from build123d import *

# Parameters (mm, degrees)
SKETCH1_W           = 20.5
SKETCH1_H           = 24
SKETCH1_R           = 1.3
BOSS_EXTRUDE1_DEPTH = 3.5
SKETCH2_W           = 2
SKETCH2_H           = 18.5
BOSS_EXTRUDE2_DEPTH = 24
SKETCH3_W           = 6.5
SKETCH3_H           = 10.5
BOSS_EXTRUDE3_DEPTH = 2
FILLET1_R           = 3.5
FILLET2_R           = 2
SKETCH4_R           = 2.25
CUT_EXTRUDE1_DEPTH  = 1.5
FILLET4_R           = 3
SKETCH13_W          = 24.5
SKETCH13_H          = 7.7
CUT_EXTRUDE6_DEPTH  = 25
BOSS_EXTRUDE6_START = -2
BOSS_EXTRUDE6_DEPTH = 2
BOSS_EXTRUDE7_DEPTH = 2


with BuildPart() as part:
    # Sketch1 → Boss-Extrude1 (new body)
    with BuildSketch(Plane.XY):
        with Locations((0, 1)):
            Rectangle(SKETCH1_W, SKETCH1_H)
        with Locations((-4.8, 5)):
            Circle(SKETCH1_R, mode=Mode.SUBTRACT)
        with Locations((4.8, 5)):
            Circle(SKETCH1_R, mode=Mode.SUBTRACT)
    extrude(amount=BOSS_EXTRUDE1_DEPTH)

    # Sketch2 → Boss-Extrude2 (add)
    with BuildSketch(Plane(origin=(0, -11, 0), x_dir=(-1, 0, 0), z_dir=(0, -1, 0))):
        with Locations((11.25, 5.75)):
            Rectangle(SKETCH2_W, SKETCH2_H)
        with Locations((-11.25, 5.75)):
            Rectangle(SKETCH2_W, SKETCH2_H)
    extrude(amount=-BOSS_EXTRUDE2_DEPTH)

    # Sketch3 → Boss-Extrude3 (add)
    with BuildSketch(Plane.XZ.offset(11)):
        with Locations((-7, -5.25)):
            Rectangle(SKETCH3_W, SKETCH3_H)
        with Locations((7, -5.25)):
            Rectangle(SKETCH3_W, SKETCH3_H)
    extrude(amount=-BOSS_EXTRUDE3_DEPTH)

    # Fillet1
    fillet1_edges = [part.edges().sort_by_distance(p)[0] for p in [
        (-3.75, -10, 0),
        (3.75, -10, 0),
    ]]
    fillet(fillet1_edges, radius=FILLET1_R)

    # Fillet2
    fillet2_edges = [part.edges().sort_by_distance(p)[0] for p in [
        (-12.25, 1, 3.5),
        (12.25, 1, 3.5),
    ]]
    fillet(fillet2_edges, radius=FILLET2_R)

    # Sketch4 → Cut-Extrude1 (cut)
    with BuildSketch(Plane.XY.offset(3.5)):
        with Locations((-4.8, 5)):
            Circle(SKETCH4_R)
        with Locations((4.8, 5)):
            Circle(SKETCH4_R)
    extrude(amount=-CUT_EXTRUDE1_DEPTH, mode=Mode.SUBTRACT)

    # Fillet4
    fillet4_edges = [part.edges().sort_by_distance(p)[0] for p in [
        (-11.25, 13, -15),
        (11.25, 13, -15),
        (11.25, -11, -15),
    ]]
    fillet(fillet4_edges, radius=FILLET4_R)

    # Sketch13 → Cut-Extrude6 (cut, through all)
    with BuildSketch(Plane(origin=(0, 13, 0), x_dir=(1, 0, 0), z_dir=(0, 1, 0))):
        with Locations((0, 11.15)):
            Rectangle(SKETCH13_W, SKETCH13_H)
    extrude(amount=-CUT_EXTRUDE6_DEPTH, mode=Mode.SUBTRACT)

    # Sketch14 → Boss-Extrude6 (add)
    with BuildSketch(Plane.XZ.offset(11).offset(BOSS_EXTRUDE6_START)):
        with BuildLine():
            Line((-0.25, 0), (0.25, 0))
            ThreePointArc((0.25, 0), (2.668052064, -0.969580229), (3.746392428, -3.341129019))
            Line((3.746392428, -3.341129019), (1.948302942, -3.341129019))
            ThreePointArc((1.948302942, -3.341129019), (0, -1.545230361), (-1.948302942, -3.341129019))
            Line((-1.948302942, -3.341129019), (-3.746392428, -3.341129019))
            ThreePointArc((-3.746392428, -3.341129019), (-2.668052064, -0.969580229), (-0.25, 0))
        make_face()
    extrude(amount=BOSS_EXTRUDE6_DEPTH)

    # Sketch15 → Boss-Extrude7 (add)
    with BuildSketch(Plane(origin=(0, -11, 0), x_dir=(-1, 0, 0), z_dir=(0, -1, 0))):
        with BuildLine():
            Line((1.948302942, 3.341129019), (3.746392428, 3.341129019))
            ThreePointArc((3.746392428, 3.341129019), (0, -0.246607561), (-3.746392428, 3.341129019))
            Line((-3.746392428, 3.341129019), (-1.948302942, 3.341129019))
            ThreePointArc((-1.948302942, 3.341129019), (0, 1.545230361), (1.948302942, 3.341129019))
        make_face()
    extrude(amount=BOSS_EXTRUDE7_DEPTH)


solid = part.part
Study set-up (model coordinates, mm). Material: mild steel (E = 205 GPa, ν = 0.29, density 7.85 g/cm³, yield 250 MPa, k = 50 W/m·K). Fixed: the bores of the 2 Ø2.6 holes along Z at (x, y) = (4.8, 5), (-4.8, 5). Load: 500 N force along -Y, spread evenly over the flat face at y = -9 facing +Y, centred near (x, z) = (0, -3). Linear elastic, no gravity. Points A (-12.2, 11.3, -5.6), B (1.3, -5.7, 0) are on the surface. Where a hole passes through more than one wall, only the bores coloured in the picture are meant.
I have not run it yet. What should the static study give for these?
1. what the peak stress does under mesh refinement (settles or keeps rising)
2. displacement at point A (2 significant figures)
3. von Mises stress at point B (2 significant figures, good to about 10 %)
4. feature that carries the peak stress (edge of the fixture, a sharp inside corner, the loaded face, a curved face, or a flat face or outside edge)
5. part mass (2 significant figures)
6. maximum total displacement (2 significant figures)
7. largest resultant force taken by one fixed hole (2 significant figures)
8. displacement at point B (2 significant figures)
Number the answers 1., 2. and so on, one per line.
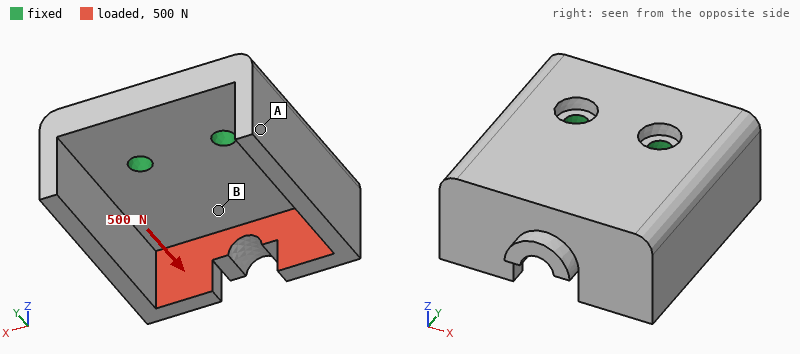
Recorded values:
1. keeps rising
2. 8.1 µm
3. 24 MPa
4. edge of the fixture
5. 23 g
6. 21 µm
7. 260 N
8. 8.1 µm
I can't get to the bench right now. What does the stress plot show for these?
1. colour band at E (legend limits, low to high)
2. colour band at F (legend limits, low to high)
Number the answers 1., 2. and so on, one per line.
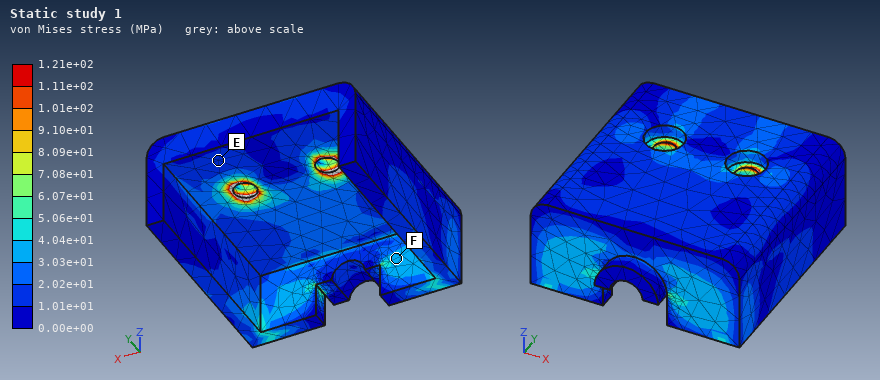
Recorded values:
1. 1.01e+01 to 2.02e+01 MPa
2. 3.03e+01 to 4.04e+01 MPa
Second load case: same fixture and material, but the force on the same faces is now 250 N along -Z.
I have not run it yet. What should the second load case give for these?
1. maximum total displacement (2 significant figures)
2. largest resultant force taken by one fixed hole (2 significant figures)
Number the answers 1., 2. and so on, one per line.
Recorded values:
1. 25 µm
2. 130 N
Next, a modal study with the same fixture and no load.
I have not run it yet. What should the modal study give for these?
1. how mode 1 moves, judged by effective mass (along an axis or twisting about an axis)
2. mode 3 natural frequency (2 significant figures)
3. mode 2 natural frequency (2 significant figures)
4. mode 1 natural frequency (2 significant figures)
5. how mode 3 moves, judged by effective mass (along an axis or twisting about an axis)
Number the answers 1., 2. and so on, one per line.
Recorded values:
1. along Z
2. 16 kHz
3. 9300 Hz
4. 6000 Hz
5. along Z
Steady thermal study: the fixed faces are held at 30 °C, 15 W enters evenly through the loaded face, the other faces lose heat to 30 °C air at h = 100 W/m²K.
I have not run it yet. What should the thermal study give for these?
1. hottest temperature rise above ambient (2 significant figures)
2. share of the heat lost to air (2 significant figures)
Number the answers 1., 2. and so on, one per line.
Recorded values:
1. 59 K
2. 33 %
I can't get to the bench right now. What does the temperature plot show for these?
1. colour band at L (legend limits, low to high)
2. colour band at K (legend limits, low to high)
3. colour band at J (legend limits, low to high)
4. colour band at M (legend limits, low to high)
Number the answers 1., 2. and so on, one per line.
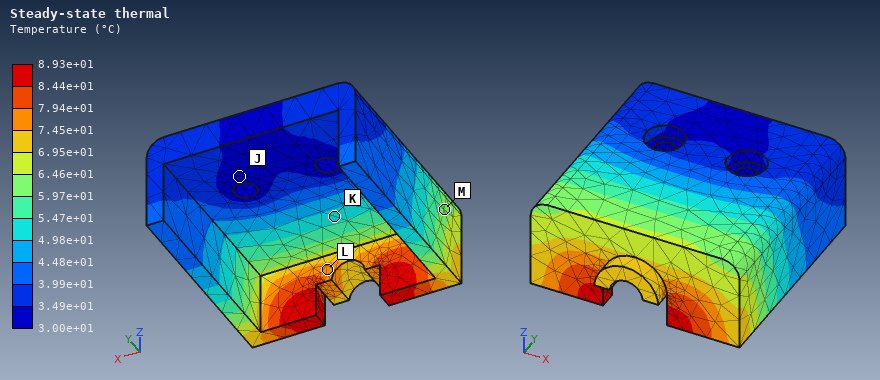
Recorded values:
1. 7.45e+01 to 7.94e+01 °C
2. 4.98e+01 to 5.47e+01 °C
3. 3.00e+01 to 3.49e+01 °C
4. 5.97e+01 to 6.46e+01 °C
